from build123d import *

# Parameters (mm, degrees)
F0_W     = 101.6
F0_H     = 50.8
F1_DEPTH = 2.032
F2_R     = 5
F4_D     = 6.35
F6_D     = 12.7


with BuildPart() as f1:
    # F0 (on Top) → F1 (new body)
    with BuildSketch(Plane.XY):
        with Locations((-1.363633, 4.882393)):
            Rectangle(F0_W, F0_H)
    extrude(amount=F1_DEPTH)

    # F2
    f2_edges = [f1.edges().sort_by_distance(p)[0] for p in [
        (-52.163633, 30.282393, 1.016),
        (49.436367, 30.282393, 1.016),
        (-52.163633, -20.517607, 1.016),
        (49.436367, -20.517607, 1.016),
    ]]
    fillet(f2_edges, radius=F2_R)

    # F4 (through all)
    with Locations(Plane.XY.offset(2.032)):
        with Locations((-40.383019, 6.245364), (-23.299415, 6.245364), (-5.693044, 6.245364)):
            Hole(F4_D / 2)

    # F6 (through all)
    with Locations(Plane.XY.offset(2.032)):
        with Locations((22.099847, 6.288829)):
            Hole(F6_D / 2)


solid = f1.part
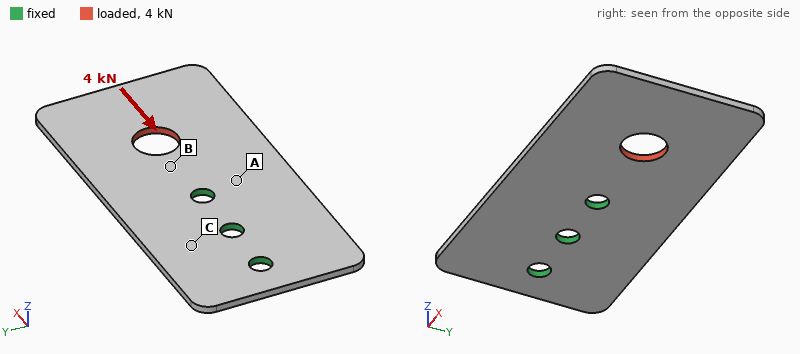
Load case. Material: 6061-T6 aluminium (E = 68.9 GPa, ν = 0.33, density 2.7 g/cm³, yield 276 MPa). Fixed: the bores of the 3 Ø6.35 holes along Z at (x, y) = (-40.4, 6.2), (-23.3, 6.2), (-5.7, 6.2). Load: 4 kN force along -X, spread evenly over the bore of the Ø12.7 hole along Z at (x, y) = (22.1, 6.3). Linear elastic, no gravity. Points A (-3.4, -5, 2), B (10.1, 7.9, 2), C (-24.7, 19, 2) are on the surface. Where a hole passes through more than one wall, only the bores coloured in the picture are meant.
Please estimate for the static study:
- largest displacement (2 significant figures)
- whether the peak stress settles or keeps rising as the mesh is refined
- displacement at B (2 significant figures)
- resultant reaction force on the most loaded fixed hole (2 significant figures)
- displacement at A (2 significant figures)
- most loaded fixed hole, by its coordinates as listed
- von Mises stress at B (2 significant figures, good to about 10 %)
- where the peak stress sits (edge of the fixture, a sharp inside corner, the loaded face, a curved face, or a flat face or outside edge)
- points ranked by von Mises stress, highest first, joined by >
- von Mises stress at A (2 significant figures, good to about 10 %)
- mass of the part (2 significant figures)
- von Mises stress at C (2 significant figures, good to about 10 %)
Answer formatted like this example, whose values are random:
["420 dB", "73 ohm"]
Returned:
["37 µm", "keeps rising", "15 µm", "2.7 kN", "9.1 µm", "(-5.7, 6.2)", "67 MPa", "edge of the fixture", "B > A > C", "29 MPa", "27 g", "16 MPa"]
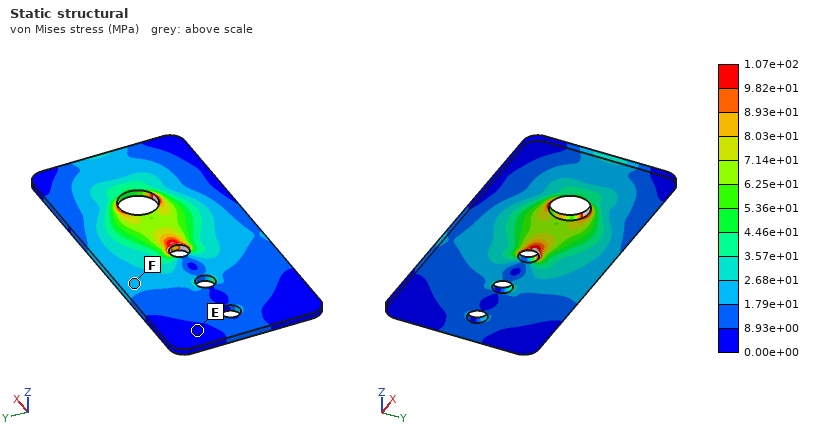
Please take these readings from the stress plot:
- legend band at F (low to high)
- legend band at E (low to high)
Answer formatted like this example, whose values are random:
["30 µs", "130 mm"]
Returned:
["1.79e+01 to 2.68e+01 MPa", "0.00e+00 to 8.93e+00 MPa"]
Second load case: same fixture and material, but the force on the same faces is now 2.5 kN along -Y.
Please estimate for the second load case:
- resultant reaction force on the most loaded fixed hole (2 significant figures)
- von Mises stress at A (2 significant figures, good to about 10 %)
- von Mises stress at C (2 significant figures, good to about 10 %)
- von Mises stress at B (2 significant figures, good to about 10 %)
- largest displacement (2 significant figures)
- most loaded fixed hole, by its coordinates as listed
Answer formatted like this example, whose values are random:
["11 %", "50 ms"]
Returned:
["4.2 kN", "55 MPa", "35 MPa", "69 MPa", "0.15 mm", "(-5.7, 6.2)"]
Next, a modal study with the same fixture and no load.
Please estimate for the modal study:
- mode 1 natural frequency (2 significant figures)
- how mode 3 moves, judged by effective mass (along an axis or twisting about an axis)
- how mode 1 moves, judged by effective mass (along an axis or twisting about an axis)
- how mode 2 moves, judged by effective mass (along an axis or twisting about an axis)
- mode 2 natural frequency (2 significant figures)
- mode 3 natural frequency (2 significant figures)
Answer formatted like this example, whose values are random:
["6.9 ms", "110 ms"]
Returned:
["540 Hz", "along Z", "along Z", "twisting about X", "1100 Hz", "2600 Hz"]
